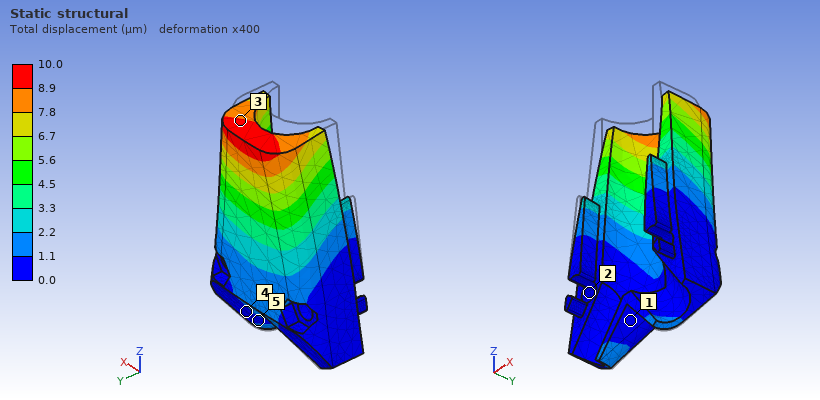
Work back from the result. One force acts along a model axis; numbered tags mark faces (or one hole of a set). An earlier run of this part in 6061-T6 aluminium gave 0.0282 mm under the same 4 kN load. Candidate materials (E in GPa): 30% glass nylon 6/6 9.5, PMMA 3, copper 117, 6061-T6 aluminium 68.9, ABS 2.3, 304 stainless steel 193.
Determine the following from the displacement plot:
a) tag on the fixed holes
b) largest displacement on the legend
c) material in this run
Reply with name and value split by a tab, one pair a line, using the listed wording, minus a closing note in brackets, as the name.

tag on the fixed holes	2
largest displacement on the legend	10.0 µm
material in this run	304 stainless steel
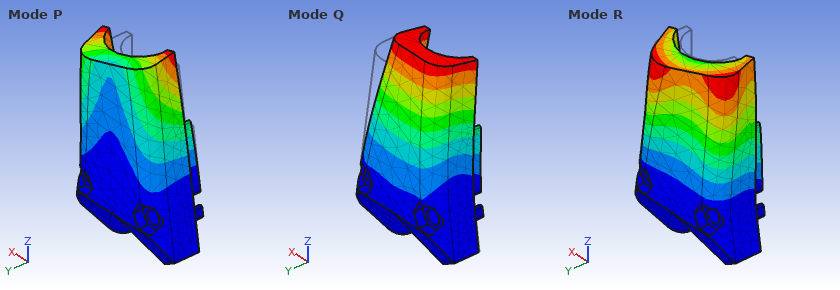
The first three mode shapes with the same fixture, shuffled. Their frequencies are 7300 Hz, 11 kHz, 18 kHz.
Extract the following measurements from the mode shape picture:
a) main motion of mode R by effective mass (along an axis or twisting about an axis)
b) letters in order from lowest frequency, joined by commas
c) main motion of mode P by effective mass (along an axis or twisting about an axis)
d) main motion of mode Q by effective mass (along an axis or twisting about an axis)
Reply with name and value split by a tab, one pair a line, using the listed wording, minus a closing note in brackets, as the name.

main motion of mode R by effective mass	along X
letters in order from lowest frequency, joined by commas	Q, P, R
main motion of mode P by effective mass	along X
main motion of mode Q by effective mass	along Y
